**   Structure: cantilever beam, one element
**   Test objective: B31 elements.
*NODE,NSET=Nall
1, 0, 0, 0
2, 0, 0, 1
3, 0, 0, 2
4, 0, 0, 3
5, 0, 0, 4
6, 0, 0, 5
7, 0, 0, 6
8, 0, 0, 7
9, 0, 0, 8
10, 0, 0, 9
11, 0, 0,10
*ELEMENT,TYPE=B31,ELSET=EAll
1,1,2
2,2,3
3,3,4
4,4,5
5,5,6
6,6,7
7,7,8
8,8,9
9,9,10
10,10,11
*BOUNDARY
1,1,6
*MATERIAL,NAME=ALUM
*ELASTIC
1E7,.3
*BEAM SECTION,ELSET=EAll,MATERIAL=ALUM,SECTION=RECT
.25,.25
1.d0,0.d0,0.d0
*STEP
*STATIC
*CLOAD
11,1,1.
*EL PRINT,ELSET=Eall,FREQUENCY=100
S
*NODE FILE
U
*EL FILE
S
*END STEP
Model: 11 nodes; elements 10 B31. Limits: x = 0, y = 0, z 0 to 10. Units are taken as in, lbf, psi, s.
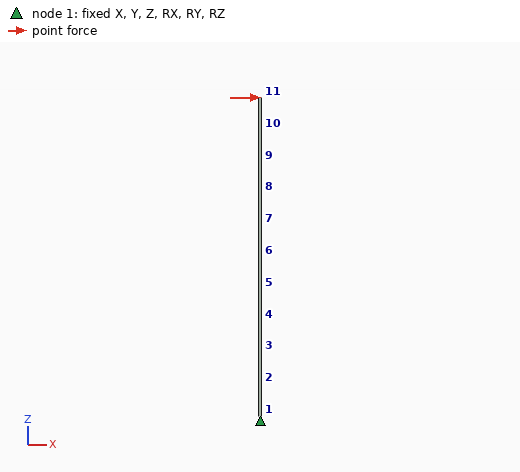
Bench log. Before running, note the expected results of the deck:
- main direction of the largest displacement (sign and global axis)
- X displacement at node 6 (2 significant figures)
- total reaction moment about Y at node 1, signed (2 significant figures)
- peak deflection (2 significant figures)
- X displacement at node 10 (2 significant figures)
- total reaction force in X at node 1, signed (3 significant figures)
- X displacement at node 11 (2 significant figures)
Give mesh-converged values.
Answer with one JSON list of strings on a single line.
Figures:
["+X", "0.032 in", "-10 lbf·in", "0.10 in", "0.087 in", "-1.00 lbf", "0.10 in"]
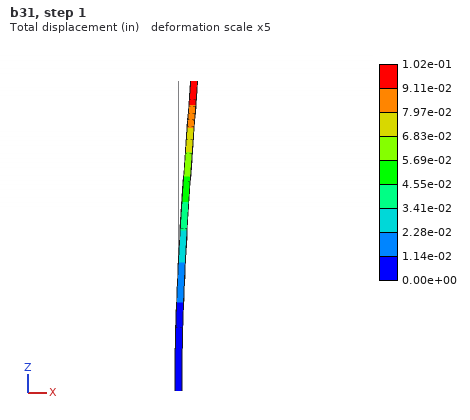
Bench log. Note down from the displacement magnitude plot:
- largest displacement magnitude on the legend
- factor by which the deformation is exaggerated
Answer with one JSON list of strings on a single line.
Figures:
["1.02e-01 in", "5"]
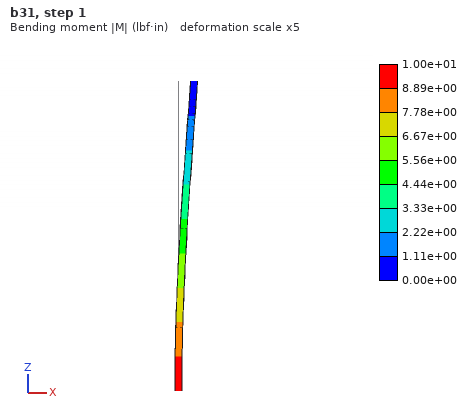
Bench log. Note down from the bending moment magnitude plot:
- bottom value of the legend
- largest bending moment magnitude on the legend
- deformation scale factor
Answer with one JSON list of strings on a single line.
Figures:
["0.00e+00 lbf·in", "1.00e+01 lbf·in", "5"]
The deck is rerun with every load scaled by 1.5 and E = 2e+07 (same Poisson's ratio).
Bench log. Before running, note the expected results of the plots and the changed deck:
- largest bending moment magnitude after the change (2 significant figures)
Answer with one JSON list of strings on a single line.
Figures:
["15 lbf·in"]
